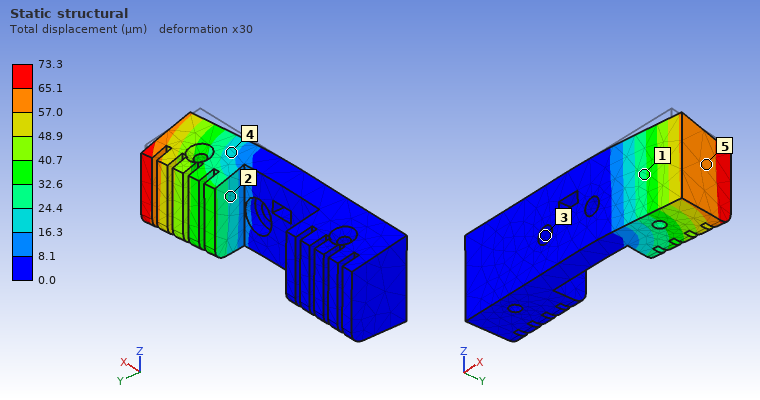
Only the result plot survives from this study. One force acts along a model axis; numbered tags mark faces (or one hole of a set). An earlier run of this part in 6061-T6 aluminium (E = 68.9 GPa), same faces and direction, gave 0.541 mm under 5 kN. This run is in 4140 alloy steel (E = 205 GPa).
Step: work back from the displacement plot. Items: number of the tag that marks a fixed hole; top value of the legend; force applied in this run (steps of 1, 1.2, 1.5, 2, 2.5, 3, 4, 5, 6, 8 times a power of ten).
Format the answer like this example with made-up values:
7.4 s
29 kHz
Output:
3
73.3 µm
2 kN
